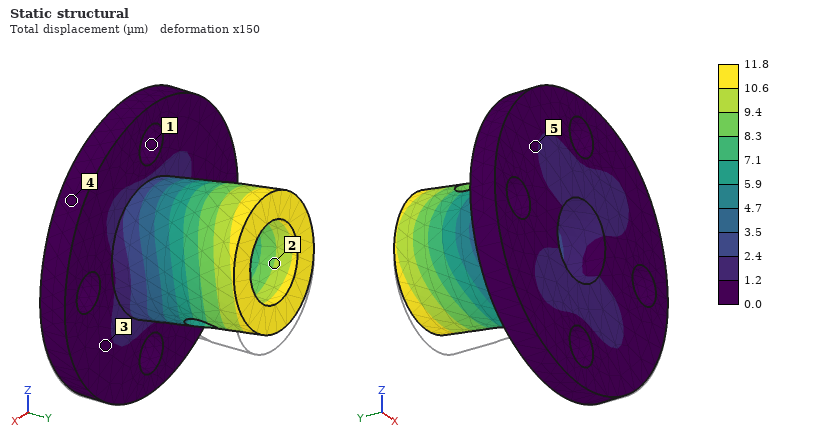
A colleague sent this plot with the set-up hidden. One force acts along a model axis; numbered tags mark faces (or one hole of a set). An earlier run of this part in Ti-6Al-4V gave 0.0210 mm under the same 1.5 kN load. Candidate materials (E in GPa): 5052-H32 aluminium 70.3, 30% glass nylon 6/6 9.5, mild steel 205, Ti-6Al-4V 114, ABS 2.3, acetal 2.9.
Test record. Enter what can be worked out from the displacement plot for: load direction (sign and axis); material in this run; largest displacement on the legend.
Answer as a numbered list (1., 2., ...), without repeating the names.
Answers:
1. +Z
2. mild steel
3. 11.8 µm
